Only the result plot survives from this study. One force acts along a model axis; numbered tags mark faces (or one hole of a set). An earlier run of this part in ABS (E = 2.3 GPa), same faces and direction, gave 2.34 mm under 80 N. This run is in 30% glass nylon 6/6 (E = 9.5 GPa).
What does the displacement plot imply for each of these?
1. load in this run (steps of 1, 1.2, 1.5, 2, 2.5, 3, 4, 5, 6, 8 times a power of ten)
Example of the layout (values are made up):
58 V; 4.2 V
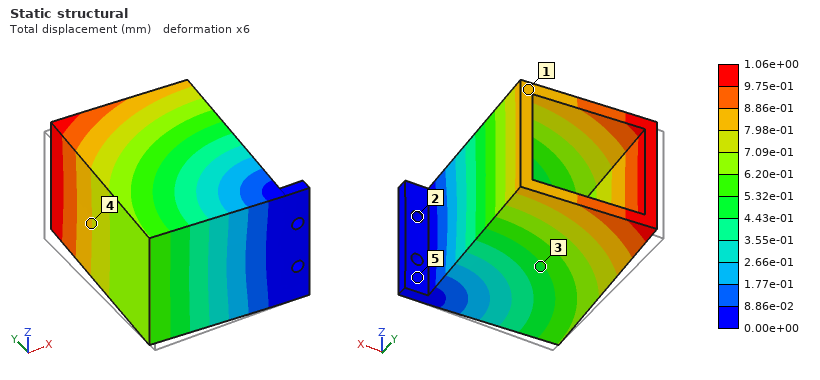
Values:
150 N
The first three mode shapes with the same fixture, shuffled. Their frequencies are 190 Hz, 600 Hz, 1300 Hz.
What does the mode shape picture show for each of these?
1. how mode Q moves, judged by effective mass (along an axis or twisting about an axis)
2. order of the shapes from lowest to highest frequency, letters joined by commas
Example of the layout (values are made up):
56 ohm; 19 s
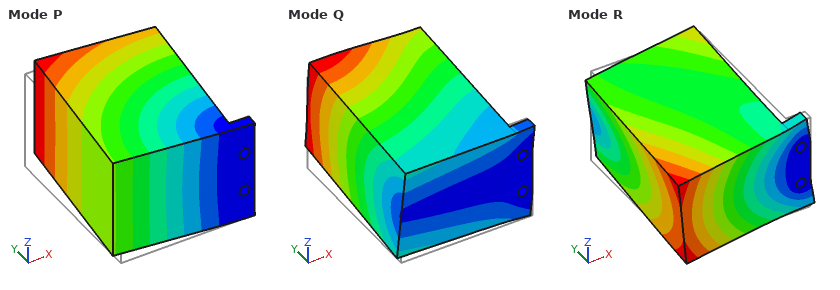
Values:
along Z; P, Q, R
